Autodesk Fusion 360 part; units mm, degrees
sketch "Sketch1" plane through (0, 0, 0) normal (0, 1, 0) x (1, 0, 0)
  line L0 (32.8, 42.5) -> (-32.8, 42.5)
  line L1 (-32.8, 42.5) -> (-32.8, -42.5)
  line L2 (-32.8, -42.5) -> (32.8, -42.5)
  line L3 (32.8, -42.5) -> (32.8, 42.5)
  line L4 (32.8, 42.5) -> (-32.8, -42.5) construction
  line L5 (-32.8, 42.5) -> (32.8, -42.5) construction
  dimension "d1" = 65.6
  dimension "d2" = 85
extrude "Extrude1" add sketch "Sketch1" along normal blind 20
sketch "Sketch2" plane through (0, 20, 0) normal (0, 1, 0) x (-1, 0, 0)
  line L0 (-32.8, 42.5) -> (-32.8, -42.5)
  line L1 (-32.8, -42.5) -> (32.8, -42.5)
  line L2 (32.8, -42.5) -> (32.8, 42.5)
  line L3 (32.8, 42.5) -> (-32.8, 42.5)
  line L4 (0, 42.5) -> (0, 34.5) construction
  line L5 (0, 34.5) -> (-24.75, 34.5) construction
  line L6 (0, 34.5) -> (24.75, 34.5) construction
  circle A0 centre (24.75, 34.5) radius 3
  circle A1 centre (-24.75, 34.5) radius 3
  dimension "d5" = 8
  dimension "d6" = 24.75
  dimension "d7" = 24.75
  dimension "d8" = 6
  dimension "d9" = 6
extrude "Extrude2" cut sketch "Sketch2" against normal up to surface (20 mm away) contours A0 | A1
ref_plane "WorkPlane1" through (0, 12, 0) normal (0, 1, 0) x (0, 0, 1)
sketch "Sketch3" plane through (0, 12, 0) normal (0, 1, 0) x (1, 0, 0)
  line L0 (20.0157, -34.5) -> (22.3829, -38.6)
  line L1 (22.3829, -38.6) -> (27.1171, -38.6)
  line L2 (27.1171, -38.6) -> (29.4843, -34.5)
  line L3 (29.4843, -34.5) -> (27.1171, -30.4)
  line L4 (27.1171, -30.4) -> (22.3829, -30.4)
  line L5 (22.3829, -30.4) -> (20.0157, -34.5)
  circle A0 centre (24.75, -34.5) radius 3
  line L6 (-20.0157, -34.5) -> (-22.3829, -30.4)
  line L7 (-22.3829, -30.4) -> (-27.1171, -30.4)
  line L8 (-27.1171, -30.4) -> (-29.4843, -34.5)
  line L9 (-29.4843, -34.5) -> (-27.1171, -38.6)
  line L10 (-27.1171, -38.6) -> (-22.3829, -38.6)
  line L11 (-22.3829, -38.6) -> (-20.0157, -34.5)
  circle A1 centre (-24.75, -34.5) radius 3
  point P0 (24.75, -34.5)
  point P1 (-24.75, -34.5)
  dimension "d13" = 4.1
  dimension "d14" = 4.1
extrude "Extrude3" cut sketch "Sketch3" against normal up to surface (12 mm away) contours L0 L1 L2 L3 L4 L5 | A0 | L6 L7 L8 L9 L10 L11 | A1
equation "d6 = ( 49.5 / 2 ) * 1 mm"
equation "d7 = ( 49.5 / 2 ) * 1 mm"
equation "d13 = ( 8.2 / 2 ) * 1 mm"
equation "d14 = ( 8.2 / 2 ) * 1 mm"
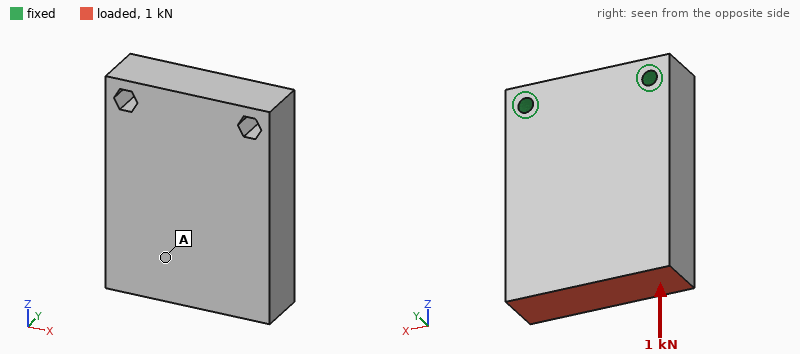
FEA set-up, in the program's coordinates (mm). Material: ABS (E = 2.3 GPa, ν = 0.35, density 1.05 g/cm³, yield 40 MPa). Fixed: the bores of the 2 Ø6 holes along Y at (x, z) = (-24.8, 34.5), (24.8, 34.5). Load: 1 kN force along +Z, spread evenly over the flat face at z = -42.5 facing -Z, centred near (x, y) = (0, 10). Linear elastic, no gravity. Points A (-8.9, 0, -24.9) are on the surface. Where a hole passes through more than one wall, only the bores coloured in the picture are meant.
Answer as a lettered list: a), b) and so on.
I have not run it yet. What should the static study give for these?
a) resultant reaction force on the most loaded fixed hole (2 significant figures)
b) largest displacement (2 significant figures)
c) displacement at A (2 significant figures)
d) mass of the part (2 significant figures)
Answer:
a) 510 N
b) 0.34 mm
c) 0.26 mm
d) 120 g
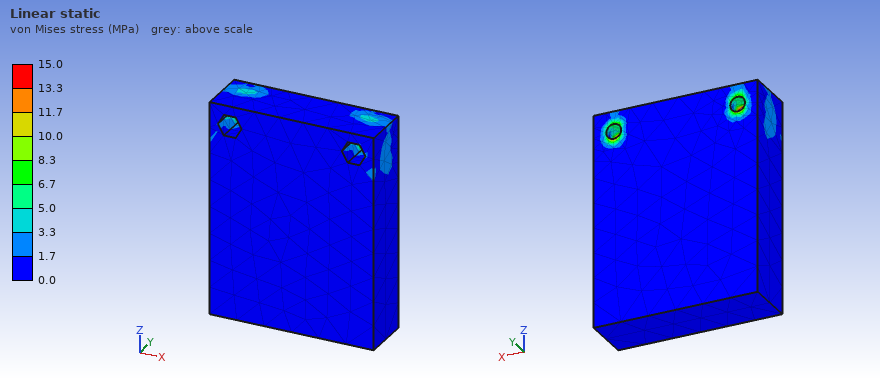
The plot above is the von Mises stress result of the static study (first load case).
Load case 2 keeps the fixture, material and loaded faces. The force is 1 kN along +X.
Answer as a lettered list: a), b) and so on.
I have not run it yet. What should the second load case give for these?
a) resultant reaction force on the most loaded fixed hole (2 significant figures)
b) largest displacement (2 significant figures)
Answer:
a) 1.6 kN
b) 0.39 mm
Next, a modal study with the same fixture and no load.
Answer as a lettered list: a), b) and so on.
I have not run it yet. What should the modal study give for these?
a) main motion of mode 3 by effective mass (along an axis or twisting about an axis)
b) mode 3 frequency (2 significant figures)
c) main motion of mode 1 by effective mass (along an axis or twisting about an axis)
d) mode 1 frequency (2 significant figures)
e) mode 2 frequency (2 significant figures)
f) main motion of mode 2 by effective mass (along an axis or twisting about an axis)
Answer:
a) along X
b) 1700 Hz
c) along Y
d) 370 Hz
e) 1400 Hz
f) along X
